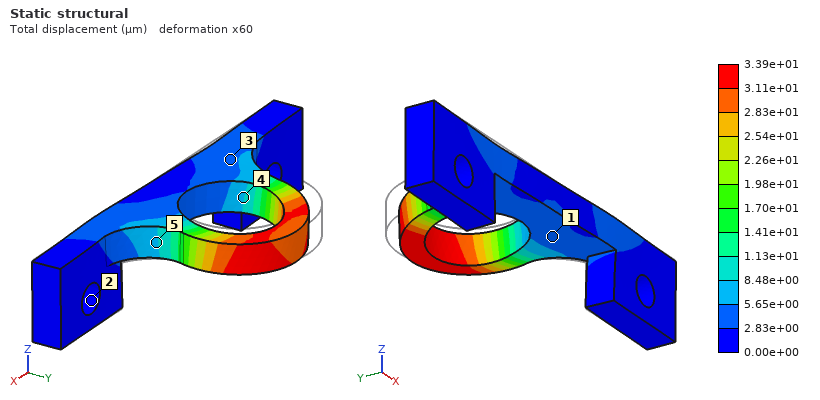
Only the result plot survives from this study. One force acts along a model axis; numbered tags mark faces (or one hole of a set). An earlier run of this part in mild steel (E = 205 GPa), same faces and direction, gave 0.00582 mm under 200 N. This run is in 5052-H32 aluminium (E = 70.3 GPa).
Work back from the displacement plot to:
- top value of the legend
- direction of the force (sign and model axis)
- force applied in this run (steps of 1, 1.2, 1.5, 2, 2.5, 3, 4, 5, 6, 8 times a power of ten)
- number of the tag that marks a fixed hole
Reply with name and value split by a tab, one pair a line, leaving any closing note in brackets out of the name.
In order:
top value of the legend	3.39e+01 µm
direction of the force	+X
force applied in this run	400 N
number of the tag that marks a fixed hole	2
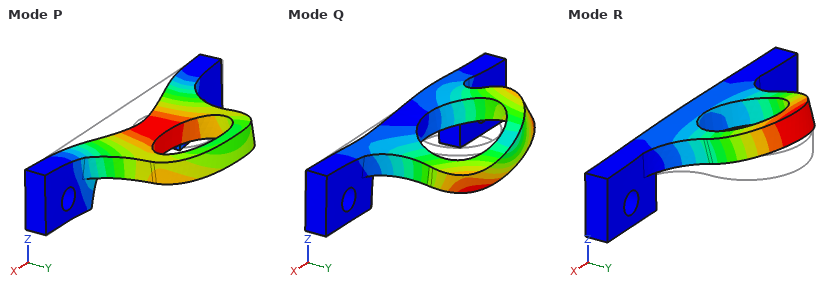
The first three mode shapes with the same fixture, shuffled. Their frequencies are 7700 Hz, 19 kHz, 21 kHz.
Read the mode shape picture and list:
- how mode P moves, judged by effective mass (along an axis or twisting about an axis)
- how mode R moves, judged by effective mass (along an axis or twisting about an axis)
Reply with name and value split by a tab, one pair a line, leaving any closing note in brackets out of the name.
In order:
how mode P moves, judged by effective mass	along Y
how mode R moves, judged by effective mass	along Z
